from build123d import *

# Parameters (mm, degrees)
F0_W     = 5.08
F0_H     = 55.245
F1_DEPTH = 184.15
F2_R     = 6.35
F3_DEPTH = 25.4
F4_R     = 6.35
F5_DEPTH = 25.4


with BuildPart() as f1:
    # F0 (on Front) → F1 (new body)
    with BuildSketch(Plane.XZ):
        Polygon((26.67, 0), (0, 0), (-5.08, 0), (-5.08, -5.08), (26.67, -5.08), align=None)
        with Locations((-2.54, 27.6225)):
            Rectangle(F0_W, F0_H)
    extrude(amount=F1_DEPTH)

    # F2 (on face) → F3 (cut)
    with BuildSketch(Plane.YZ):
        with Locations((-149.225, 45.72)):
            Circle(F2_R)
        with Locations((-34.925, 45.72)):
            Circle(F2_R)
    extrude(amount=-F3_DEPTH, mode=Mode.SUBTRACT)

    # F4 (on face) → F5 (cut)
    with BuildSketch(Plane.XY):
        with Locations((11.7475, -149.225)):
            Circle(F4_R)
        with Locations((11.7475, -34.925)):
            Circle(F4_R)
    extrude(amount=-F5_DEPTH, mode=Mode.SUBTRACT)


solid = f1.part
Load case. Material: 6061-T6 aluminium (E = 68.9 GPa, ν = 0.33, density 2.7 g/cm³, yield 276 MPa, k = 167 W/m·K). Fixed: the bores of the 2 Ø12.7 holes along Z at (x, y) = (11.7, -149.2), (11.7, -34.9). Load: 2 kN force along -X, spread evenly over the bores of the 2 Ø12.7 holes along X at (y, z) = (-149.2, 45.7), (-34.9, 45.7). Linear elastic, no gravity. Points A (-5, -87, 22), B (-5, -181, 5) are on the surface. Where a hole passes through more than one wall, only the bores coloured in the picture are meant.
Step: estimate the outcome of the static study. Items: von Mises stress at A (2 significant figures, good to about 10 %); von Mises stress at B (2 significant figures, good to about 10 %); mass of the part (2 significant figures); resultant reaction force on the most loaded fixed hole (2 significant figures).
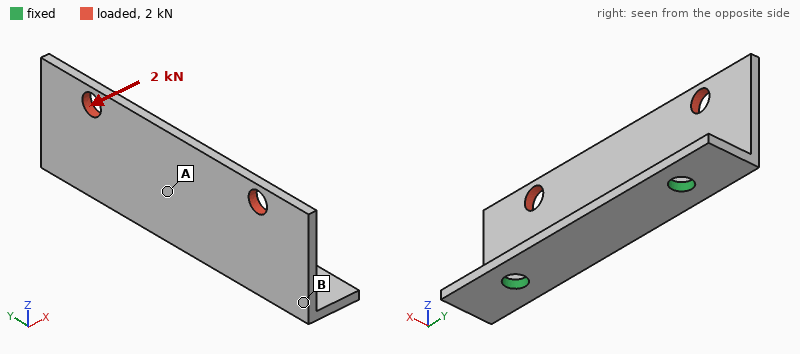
40 MPa
100 MPa
210 g
1.0 kN
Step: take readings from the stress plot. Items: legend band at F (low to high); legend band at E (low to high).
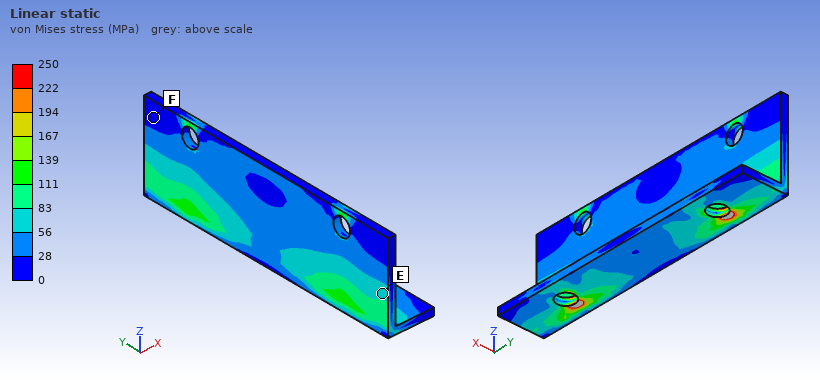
0 to 28 MPa
56 to 83 MPa
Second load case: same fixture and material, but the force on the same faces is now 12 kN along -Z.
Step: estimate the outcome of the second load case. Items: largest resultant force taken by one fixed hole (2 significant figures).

6.0 kN
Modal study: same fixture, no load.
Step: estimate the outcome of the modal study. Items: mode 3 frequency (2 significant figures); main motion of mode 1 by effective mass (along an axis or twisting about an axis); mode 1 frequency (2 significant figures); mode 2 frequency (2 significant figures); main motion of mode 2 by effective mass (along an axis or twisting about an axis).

2000 Hz
along X
890 Hz
1300 Hz
twisting about Z
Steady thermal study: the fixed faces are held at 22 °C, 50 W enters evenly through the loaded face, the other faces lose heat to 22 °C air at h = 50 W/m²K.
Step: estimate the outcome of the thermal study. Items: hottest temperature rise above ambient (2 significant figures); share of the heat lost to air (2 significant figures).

29 K
32 %
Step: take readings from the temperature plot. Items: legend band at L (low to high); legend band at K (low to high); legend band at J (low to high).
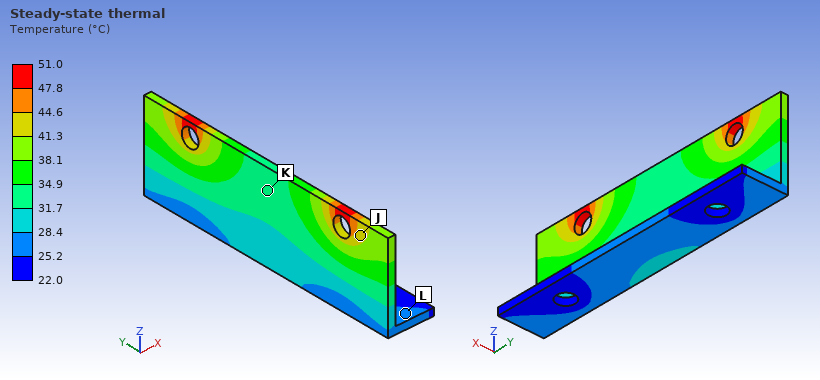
25.2 to 28.4 °C
31.7 to 34.9 °C
41.3 to 44.6 °C
